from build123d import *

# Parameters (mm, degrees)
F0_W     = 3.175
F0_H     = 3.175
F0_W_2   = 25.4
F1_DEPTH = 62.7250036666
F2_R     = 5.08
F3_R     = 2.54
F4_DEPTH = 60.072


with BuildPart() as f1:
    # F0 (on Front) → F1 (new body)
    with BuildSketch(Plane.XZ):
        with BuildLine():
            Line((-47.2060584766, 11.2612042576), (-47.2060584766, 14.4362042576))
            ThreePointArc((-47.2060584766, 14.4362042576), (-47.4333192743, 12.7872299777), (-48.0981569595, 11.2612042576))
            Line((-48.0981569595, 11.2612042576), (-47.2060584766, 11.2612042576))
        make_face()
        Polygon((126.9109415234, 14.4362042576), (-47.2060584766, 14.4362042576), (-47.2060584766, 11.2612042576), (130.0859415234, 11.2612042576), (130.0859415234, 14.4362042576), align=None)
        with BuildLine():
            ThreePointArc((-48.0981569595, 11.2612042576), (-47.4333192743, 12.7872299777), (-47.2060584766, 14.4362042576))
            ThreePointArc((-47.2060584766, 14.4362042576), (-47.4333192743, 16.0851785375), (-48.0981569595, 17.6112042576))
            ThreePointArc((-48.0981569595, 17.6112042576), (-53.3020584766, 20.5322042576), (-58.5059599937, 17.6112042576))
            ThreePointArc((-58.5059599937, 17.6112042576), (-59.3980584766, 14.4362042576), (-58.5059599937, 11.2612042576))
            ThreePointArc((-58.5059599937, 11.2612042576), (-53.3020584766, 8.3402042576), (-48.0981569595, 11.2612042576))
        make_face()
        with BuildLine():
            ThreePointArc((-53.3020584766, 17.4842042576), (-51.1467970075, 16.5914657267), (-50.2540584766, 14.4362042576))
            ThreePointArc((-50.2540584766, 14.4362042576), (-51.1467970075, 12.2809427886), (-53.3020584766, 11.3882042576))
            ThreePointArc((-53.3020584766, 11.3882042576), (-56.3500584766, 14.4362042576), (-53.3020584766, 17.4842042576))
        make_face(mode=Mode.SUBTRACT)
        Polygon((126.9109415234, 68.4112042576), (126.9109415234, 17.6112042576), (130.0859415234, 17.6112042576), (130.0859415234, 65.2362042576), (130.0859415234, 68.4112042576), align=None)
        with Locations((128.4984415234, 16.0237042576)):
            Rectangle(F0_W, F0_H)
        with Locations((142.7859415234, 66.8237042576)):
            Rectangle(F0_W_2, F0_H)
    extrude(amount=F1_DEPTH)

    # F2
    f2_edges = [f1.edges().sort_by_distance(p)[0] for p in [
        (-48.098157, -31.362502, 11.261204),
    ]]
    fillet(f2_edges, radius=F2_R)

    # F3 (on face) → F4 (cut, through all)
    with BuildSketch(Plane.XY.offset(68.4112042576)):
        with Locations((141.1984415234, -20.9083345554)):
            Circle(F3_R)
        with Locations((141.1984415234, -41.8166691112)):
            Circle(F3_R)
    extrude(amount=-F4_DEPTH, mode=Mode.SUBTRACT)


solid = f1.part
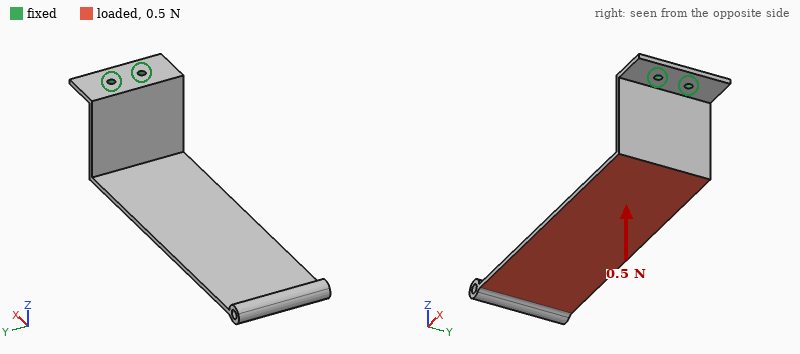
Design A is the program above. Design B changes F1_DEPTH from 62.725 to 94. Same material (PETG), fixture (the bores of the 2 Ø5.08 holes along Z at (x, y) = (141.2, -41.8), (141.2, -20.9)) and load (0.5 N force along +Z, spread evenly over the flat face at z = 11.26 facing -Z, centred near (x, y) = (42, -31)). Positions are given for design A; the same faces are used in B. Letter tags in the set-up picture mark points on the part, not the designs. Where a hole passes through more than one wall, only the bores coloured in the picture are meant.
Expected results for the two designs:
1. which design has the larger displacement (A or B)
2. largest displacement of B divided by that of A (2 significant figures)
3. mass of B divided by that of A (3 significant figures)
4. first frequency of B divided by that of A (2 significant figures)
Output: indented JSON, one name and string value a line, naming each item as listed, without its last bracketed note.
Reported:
{
  "which design has the larger displacement": "A",
  "largest displacement of B divided by that of A": "0.71",
  "mass of B divided by that of A": "1.50",
  "first frequency of B divided by that of A": "0.97"
}
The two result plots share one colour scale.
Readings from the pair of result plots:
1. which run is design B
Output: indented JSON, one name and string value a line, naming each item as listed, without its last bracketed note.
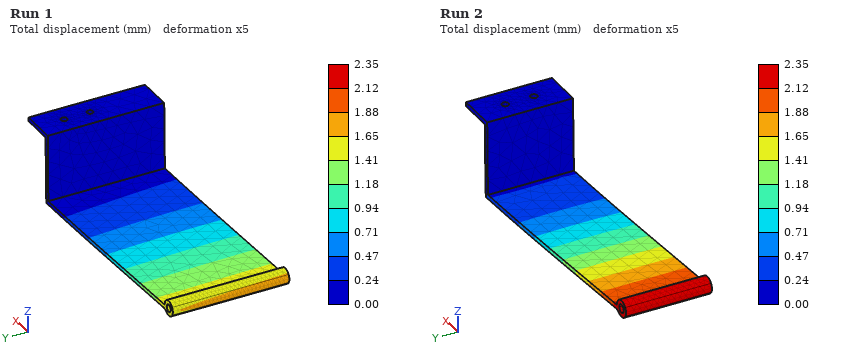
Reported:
{
  "which run is design B": "Run 1"
}
